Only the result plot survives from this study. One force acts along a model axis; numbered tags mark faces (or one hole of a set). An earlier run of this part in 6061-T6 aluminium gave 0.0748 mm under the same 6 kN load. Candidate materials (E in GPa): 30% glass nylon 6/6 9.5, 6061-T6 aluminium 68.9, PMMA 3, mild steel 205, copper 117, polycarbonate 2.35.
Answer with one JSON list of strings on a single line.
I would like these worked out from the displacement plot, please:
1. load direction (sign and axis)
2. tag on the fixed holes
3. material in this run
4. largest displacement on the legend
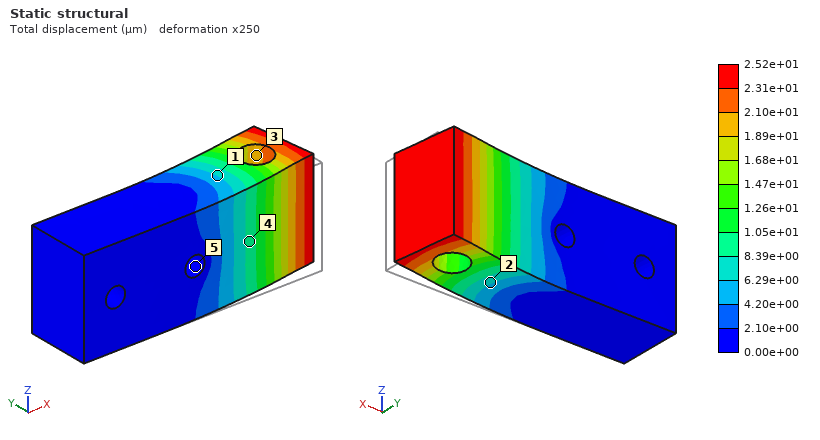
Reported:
["+Y", "5", "mild steel", "2.52e+01 µm"]
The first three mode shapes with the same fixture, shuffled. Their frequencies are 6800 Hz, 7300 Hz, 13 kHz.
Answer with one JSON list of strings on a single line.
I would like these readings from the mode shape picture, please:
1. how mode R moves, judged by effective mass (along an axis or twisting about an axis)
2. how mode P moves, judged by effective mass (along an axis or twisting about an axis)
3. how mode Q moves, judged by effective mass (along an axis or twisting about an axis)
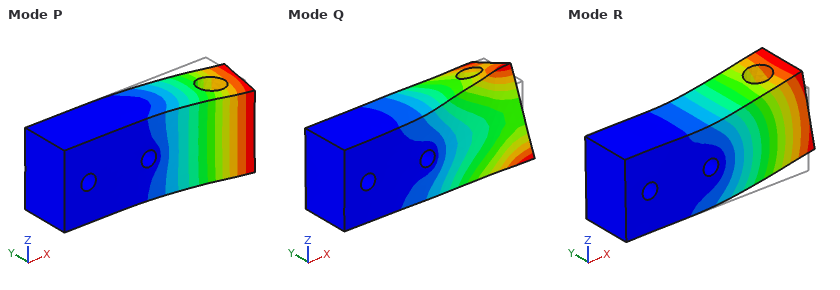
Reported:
["along Z", "along Y", "twisting about X"]
